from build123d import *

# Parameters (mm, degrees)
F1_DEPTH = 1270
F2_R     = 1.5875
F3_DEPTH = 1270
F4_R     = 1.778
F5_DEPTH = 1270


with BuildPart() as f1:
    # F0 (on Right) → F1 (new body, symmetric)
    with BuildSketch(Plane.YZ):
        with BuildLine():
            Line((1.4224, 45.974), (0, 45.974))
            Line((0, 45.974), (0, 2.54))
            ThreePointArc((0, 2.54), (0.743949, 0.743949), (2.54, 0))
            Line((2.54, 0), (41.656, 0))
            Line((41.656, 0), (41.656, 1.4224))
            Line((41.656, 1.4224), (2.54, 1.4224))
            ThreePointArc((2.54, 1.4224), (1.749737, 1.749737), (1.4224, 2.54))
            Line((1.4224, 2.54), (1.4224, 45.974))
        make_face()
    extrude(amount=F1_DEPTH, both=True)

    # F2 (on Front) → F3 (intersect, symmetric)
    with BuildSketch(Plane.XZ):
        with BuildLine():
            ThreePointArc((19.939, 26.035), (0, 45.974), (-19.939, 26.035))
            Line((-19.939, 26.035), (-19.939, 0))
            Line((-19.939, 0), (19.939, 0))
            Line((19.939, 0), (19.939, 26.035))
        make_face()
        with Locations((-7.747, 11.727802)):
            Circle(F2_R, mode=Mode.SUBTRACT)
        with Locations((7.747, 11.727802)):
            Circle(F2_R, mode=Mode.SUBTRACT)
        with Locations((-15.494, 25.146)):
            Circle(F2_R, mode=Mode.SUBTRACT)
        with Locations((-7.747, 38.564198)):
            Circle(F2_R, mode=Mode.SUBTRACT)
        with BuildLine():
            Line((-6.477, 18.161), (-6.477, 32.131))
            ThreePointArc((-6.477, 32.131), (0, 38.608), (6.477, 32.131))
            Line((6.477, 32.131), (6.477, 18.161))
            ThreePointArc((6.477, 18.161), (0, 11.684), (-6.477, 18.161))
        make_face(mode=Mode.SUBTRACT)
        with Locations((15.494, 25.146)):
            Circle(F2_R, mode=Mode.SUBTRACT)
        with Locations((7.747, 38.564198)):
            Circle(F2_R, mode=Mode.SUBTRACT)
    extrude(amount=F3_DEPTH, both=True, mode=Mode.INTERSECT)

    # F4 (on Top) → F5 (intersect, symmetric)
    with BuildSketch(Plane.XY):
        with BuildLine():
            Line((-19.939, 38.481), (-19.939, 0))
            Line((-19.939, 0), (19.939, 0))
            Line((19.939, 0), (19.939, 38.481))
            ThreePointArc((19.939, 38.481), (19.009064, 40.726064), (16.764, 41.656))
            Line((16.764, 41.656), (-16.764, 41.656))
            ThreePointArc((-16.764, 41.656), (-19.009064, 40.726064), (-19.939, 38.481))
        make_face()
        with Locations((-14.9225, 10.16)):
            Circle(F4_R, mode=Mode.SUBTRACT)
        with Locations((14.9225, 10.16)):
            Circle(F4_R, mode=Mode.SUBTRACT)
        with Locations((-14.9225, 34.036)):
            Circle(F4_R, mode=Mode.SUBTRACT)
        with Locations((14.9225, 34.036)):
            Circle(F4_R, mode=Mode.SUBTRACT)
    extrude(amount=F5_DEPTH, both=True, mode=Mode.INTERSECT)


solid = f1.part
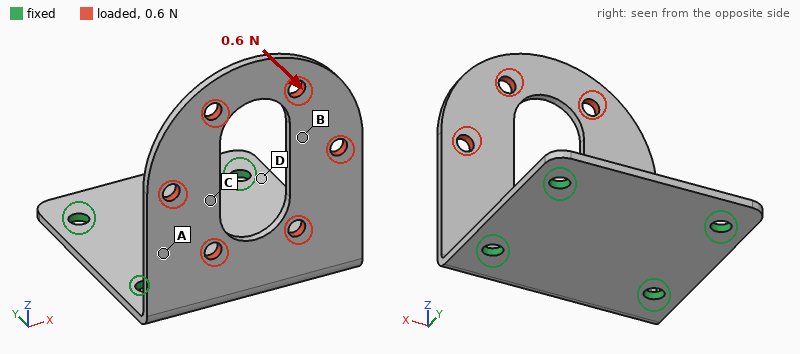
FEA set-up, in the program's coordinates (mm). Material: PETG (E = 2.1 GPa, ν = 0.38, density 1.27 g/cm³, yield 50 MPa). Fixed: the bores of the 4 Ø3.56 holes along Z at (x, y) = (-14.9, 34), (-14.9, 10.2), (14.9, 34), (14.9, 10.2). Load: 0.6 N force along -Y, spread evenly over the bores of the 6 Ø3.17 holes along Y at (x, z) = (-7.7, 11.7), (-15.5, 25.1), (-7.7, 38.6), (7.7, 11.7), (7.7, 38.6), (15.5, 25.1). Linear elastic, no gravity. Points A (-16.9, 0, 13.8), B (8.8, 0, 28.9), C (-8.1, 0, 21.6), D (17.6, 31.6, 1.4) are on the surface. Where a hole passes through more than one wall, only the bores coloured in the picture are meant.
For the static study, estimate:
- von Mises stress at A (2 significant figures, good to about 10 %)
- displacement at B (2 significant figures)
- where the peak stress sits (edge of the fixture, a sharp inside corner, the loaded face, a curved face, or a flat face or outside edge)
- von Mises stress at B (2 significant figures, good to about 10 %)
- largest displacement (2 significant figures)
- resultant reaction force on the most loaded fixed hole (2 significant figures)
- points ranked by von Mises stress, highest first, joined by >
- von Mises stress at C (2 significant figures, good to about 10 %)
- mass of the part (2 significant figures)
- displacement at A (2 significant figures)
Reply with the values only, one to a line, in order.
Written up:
0.73 MPa
0.36 mm
a flat face or outside edge
0.28 MPa
0.69 mm
0.21 N
A > C > B > D
0.51 MPa
5.1 g
0.13 mm
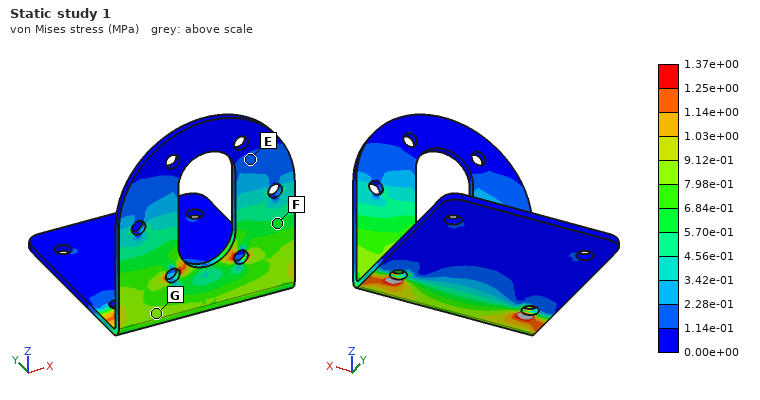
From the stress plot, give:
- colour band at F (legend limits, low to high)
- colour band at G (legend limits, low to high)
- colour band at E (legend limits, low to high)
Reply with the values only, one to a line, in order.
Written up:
5.70e-01 to 6.84e-01 MPa
7.98e-01 to 9.12e-01 MPa
1.14e-01 to 2.28e-01 MPa
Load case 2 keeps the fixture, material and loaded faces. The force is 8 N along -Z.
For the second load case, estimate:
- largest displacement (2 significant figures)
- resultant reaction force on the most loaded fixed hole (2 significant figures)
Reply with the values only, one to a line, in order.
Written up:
0.71 mm
4.2 N
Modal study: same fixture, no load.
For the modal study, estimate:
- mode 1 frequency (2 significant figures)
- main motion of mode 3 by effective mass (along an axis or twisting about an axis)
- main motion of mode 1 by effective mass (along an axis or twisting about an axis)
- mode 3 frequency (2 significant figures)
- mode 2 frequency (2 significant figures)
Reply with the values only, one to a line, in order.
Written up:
140 Hz
along X
along Y
660 Hz
380 Hz
